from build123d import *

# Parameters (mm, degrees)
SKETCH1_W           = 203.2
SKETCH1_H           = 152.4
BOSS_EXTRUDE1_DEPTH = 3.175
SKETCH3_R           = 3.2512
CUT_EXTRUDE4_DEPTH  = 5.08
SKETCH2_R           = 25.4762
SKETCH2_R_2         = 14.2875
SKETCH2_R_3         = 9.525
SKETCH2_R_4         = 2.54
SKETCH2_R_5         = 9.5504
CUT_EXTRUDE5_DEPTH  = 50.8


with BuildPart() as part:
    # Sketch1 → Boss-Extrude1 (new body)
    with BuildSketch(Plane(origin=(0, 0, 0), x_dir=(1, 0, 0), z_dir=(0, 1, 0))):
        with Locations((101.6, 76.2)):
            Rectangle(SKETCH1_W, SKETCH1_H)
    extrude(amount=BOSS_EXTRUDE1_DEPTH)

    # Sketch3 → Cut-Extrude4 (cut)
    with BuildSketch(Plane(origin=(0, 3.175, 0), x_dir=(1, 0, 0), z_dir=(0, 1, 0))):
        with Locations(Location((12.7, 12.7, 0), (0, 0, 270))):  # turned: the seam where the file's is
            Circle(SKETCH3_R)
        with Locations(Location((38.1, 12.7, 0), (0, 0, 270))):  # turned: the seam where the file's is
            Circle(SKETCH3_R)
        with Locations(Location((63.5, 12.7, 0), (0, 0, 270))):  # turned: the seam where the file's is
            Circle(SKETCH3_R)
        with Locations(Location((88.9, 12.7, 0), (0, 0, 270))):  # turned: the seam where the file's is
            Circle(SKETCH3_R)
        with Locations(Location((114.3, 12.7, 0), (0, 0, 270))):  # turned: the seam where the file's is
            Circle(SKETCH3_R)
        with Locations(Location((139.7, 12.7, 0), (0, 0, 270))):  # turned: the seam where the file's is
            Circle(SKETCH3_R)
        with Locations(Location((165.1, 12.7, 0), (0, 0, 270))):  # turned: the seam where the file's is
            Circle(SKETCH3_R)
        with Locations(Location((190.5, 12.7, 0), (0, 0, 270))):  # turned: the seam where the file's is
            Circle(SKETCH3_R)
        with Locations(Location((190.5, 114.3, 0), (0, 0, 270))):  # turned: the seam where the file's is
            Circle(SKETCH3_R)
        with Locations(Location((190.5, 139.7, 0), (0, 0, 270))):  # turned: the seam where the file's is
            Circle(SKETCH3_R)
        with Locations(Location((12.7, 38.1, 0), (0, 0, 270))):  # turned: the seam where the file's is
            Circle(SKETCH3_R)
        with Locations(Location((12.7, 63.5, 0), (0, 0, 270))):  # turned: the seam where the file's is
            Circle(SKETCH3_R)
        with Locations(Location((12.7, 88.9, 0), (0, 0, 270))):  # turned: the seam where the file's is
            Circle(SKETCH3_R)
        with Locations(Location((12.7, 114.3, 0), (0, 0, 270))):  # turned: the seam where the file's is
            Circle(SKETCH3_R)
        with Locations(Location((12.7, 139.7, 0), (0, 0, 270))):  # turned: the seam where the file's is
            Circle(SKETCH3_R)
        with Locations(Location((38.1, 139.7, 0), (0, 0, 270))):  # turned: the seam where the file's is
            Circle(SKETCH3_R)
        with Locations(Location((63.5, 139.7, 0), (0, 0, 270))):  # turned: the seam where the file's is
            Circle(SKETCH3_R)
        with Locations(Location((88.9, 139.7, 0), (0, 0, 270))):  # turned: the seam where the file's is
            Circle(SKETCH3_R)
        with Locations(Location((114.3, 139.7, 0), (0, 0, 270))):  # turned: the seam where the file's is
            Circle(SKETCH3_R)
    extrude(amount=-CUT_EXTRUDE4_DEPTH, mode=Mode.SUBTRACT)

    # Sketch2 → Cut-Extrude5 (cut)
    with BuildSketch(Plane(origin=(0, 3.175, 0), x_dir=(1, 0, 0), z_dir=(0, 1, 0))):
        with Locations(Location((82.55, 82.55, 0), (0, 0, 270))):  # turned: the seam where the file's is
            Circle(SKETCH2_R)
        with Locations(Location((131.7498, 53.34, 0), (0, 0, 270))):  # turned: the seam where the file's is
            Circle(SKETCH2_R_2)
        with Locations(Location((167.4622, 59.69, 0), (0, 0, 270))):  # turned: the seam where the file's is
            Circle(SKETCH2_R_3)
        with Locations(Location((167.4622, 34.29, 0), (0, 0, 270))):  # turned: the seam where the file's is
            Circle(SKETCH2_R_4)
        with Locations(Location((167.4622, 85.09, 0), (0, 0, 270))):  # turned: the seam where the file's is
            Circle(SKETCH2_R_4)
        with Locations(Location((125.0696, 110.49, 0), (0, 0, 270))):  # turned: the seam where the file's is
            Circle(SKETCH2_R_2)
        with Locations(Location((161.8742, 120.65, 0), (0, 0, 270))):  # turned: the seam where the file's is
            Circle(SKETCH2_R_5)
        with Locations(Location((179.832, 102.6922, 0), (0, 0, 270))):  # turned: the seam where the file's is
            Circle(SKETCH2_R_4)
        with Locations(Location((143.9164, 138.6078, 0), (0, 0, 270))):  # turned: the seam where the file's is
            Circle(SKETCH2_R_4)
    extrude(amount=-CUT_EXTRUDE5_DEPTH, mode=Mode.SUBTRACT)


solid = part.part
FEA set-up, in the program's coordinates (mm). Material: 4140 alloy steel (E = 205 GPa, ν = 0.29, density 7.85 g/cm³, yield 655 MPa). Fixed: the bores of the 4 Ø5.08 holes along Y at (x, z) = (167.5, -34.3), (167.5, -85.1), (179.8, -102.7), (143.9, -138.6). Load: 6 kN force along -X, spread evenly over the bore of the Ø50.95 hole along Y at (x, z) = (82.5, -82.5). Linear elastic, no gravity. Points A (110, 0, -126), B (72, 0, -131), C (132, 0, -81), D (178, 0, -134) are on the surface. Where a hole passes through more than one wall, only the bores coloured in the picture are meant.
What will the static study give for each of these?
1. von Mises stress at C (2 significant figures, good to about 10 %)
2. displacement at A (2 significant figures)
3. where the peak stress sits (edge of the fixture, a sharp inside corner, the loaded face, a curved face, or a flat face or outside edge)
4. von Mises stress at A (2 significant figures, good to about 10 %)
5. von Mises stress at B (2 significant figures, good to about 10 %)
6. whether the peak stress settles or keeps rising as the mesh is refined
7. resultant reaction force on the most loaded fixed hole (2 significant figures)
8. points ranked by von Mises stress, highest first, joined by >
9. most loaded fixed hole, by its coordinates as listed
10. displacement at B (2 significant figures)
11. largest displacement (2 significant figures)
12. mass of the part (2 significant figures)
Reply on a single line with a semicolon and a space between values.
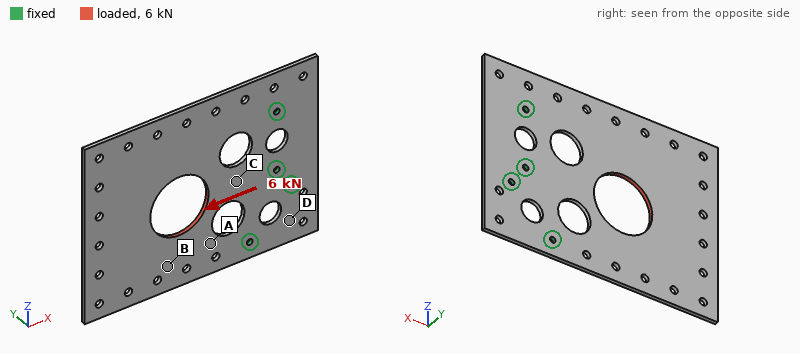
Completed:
17 MPa; 5.4 µm; edge of the fixture; 28 MPa; 9.7 MPa; keeps rising; 2.5 kN; A > C > B > D; (167.5, -34.3); 7.8 µm; 14 µm; 660 g
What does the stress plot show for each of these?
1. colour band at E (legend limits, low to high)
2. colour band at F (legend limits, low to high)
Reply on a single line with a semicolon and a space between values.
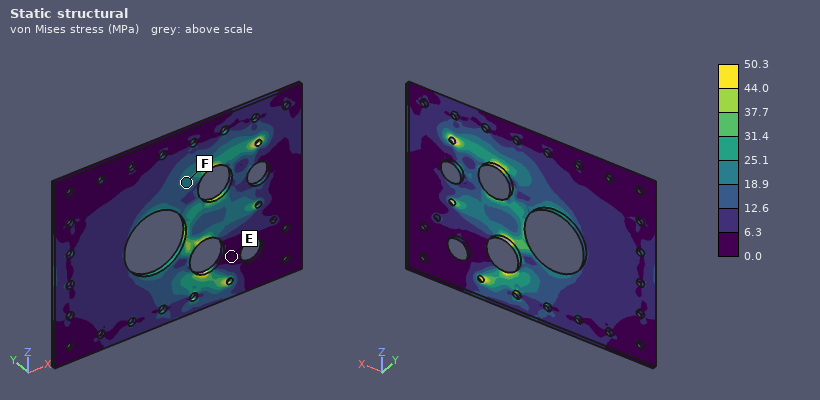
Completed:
0.0 to 6.3 MPa; 18.9 to 25.1 MPa
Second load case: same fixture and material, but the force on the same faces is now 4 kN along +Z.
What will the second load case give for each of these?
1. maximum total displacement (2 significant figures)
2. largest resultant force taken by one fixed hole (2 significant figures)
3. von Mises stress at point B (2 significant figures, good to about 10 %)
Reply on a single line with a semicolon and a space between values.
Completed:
43 µm; 3.2 kN; 8.8 MPa
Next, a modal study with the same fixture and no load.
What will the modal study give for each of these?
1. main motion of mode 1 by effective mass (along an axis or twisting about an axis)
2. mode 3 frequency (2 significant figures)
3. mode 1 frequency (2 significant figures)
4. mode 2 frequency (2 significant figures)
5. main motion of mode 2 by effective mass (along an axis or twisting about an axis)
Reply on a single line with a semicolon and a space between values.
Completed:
along Y; 600 Hz; 90 Hz; 240 Hz; twisting about X
